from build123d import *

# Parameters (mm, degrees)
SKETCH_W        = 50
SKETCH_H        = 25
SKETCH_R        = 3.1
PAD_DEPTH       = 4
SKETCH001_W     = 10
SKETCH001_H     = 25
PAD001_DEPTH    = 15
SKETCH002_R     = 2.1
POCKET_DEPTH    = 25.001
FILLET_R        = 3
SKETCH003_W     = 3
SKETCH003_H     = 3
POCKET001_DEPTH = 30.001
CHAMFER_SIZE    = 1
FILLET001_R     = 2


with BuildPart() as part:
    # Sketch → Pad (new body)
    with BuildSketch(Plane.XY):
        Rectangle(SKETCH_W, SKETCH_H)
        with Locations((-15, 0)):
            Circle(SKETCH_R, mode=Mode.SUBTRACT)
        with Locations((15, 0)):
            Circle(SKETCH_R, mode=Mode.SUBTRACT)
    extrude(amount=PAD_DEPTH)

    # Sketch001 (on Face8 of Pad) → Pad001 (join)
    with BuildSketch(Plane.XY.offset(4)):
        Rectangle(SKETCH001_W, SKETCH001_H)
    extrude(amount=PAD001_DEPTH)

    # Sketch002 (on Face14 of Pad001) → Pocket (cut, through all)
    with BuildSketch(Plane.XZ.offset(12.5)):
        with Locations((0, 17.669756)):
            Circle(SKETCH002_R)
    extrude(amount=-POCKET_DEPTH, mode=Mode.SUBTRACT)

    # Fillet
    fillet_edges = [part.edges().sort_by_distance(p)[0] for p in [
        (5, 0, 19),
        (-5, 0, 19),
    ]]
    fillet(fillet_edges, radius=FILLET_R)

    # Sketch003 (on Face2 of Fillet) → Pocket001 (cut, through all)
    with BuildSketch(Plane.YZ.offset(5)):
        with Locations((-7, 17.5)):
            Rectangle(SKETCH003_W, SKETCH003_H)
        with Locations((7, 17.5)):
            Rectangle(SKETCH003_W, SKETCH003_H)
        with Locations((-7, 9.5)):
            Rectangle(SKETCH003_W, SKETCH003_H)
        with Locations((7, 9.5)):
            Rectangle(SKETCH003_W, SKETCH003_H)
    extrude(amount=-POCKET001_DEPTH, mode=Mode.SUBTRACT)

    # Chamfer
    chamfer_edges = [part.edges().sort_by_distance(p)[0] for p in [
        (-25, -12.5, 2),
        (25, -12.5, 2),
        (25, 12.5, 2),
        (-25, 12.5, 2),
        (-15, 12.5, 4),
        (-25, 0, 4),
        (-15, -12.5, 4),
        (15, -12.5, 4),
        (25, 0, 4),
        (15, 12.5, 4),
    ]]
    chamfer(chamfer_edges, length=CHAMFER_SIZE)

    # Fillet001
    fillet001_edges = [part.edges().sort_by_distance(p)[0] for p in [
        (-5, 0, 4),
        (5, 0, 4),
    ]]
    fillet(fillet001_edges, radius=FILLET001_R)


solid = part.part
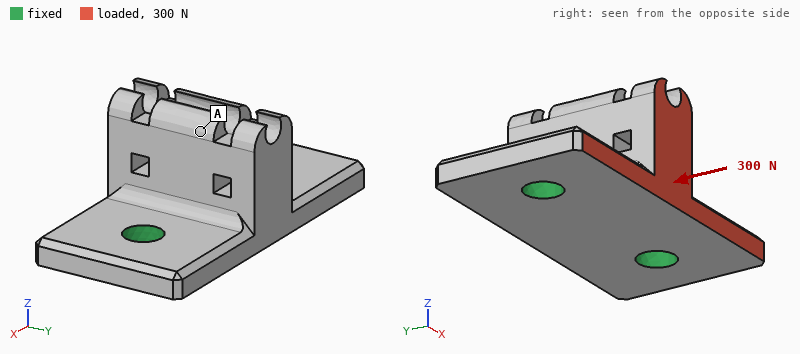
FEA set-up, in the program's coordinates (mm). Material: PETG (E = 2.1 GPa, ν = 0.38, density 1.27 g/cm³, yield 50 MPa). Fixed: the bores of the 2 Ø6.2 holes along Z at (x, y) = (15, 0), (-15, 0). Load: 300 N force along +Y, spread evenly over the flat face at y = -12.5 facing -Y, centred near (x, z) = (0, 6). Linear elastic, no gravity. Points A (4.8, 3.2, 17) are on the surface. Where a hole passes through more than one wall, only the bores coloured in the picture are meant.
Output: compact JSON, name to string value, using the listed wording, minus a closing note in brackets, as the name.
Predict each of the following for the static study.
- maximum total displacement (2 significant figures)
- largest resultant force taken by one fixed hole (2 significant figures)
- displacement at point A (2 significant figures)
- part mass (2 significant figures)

{"maximum total displacement": "0.23 mm", "largest resultant force taken by one fixed hole": "150 N", "displacement at point A": "0.17 mm", "part mass": "9.9 g"}
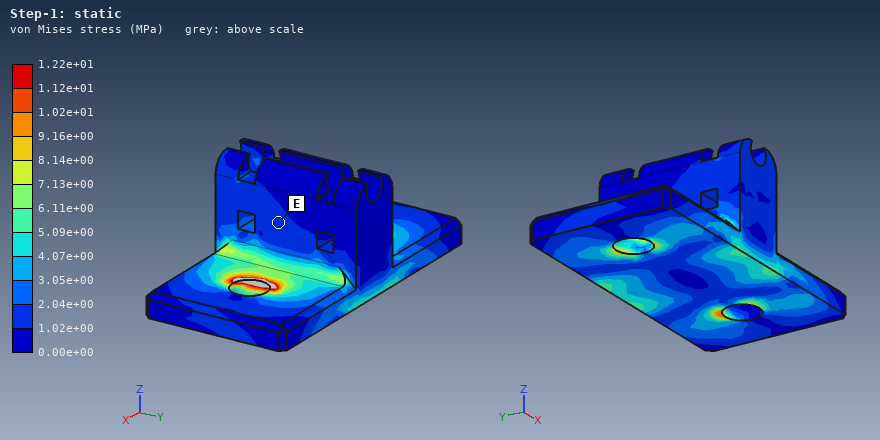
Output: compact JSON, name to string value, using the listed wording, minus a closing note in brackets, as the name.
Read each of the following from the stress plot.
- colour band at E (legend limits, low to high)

{"colour band at E": "1.02e+00 to 2.04e+00 MPa"}
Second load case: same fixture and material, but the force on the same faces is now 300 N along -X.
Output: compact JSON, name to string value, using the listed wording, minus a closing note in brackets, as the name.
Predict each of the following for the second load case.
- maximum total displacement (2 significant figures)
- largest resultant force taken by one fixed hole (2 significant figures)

{"maximum total displacement": "0.15 mm", "largest resultant force taken by one fixed hole": "190 N"}
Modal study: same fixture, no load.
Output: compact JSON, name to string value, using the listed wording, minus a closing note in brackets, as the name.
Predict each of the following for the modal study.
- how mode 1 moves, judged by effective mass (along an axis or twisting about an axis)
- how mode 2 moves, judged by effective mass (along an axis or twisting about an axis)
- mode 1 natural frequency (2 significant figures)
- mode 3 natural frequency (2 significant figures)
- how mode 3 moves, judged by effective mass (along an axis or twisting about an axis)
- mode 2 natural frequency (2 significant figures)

{"how mode 1 moves, judged by effective mass": "along Y", "how mode 2 moves, judged by effective mass": "along Z", "mode 1 natural frequency": "2100 Hz", "mode 3 natural frequency": "4300 Hz", "how mode 3 moves, judged by effective mass": "along X", "mode 2 natural frequency": "4000 Hz"}
